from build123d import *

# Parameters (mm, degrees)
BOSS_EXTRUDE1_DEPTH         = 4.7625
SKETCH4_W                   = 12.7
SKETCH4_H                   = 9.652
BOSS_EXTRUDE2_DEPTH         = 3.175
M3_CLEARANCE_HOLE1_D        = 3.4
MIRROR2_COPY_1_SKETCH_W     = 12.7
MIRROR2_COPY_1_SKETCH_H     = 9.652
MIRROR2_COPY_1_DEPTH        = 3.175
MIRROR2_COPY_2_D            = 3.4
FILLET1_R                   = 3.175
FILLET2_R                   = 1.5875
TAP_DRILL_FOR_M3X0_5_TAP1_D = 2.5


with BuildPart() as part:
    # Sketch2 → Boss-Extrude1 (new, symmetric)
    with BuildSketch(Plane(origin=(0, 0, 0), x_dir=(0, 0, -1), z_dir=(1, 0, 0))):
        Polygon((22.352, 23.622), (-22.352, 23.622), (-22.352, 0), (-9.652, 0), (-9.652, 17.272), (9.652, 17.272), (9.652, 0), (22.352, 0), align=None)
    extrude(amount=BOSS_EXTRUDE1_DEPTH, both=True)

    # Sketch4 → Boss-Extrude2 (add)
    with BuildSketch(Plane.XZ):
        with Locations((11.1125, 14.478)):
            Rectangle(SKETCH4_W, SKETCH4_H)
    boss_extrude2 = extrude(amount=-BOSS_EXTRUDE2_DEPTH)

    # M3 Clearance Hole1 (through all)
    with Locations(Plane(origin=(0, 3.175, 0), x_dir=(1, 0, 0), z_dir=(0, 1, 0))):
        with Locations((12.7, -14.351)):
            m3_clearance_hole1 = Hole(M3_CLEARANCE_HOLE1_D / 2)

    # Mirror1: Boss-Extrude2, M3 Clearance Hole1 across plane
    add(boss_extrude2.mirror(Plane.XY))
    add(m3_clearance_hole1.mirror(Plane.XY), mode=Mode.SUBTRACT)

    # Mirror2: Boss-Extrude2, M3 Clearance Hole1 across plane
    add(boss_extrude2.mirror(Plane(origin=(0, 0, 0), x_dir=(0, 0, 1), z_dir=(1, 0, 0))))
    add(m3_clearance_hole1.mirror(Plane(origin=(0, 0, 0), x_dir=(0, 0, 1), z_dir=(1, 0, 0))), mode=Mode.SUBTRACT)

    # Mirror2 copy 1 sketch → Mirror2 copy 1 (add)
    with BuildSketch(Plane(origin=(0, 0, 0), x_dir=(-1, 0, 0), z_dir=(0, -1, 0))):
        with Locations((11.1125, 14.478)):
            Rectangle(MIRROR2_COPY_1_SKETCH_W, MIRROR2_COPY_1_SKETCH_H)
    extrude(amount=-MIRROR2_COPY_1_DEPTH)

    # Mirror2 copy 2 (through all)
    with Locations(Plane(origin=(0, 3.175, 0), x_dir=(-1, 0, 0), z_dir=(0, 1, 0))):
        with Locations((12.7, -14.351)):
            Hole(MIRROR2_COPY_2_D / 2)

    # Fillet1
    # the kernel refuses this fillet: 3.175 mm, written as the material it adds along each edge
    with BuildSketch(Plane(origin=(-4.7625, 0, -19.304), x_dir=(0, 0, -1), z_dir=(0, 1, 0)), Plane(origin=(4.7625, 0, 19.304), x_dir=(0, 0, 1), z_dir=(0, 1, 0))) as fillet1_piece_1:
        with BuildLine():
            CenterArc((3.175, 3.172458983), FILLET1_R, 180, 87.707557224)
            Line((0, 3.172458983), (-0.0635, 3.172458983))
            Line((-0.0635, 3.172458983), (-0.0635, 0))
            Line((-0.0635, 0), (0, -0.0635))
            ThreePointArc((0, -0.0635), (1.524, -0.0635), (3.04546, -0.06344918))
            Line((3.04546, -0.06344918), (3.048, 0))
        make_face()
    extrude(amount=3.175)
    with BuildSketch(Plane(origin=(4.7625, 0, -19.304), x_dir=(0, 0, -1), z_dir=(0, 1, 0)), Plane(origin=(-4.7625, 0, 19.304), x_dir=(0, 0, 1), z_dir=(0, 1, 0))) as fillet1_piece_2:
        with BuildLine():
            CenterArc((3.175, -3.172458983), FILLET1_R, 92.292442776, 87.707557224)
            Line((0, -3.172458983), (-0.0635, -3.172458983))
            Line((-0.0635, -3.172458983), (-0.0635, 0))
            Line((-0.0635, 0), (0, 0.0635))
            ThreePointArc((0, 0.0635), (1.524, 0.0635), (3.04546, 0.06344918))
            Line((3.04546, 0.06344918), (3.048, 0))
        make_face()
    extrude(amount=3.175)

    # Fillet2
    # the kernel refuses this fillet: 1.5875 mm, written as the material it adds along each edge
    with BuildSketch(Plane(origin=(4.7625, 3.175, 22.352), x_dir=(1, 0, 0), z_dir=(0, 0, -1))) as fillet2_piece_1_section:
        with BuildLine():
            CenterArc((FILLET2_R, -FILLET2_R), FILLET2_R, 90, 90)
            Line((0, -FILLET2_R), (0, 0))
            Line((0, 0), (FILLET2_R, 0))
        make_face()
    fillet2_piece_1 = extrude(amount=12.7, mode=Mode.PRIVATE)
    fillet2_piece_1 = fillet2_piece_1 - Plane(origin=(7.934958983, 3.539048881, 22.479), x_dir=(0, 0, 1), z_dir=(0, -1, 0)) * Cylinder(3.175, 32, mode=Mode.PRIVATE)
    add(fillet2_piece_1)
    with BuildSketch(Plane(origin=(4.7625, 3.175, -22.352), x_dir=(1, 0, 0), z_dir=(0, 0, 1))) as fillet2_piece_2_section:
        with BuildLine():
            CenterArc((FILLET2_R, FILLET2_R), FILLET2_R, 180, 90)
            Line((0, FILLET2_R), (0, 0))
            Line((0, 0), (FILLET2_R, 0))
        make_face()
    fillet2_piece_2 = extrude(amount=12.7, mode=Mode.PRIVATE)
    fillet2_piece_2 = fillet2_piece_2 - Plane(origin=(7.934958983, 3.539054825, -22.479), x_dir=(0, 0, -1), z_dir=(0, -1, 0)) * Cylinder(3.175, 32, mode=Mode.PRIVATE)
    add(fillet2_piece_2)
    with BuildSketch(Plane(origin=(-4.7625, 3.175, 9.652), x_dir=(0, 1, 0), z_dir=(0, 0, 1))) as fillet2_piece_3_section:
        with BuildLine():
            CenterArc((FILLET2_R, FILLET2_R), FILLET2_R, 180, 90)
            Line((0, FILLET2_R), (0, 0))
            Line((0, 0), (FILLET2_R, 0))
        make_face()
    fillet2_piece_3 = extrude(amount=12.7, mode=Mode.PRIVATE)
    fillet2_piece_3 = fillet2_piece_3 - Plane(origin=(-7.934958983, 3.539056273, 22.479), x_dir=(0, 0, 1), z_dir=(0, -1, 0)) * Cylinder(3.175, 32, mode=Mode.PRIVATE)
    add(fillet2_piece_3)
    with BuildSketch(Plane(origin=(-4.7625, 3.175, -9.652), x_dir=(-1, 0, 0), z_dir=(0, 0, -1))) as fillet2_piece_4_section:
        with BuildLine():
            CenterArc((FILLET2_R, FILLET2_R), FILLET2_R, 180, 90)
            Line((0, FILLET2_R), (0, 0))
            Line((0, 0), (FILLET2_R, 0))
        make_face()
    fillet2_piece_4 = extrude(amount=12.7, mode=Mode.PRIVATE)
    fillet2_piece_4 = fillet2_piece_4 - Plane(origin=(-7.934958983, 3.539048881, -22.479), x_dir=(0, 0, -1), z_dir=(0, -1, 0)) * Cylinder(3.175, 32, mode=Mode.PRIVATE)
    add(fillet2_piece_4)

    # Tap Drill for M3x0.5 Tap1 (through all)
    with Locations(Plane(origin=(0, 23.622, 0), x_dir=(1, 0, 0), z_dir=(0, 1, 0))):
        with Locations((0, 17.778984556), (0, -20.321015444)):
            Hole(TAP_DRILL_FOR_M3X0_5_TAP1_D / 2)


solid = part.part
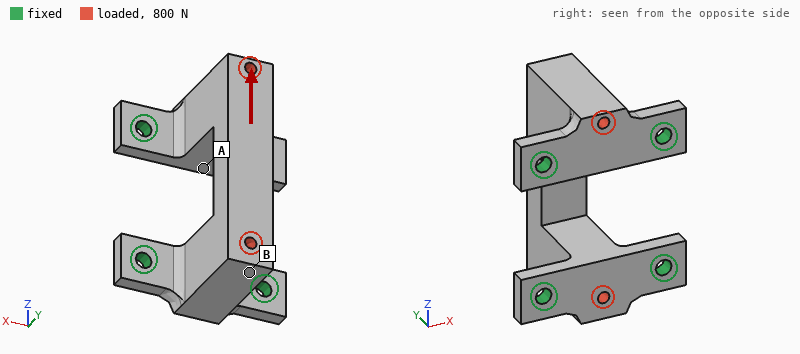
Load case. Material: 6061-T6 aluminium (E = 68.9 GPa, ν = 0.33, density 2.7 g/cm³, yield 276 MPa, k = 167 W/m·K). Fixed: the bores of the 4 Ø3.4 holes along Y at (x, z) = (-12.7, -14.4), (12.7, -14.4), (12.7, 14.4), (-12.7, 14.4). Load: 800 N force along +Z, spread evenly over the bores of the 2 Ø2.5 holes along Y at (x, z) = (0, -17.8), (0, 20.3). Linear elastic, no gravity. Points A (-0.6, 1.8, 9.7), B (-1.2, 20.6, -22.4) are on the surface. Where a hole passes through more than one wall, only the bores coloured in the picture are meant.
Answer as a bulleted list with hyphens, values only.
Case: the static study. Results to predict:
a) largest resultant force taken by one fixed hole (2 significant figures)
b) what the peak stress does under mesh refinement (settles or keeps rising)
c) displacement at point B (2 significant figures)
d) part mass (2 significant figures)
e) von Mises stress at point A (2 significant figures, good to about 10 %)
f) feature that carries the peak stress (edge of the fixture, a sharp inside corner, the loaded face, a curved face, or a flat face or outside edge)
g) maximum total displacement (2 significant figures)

- 230 N
- keeps rising
- 31 µm
- 22 g
- 12 MPa
- edge of the fixture
- 35 µm
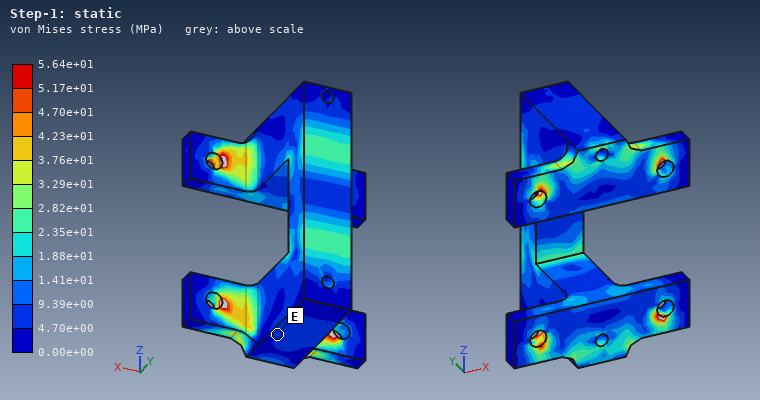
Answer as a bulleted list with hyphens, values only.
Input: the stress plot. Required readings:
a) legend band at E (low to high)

- 4.70e+00 to 9.39e+00 MPa
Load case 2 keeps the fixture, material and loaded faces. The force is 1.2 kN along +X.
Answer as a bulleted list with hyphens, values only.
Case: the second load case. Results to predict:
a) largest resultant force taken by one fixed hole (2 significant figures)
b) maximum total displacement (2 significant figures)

- 480 N
- 46 µm
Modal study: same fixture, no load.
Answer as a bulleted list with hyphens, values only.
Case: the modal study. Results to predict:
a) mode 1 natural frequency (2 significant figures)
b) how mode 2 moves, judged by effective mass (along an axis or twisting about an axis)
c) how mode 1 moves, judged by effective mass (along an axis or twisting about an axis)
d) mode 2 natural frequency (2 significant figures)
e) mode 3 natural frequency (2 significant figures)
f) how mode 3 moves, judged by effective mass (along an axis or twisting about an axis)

- 6100 Hz
- along X
- along Z
- 6900 Hz
- 12 kHz
- twisting about Y
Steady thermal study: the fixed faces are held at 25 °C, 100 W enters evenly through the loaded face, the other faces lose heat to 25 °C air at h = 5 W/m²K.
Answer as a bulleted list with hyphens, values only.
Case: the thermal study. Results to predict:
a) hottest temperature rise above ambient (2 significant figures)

- 71 K
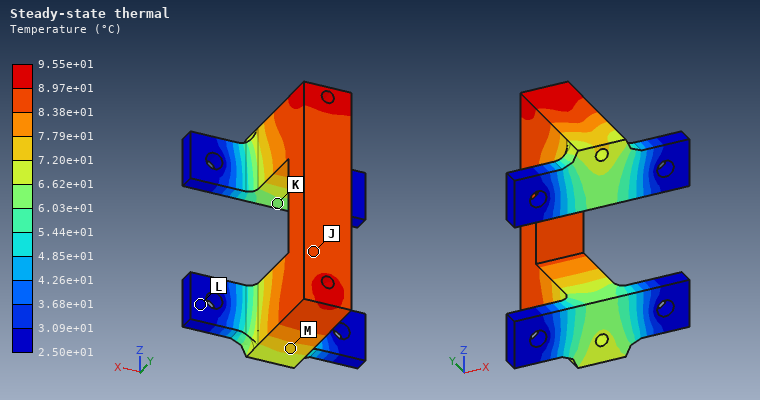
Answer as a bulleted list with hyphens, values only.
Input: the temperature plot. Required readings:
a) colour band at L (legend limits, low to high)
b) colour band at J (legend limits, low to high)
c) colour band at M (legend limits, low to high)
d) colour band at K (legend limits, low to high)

- 2.50e+01 to 3.09e+01 °C
- 8.38e+01 to 8.97e+01 °C
- 7.20e+01 to 7.79e+01 °C
- 6.03e+01 to 6.62e+01 °C
